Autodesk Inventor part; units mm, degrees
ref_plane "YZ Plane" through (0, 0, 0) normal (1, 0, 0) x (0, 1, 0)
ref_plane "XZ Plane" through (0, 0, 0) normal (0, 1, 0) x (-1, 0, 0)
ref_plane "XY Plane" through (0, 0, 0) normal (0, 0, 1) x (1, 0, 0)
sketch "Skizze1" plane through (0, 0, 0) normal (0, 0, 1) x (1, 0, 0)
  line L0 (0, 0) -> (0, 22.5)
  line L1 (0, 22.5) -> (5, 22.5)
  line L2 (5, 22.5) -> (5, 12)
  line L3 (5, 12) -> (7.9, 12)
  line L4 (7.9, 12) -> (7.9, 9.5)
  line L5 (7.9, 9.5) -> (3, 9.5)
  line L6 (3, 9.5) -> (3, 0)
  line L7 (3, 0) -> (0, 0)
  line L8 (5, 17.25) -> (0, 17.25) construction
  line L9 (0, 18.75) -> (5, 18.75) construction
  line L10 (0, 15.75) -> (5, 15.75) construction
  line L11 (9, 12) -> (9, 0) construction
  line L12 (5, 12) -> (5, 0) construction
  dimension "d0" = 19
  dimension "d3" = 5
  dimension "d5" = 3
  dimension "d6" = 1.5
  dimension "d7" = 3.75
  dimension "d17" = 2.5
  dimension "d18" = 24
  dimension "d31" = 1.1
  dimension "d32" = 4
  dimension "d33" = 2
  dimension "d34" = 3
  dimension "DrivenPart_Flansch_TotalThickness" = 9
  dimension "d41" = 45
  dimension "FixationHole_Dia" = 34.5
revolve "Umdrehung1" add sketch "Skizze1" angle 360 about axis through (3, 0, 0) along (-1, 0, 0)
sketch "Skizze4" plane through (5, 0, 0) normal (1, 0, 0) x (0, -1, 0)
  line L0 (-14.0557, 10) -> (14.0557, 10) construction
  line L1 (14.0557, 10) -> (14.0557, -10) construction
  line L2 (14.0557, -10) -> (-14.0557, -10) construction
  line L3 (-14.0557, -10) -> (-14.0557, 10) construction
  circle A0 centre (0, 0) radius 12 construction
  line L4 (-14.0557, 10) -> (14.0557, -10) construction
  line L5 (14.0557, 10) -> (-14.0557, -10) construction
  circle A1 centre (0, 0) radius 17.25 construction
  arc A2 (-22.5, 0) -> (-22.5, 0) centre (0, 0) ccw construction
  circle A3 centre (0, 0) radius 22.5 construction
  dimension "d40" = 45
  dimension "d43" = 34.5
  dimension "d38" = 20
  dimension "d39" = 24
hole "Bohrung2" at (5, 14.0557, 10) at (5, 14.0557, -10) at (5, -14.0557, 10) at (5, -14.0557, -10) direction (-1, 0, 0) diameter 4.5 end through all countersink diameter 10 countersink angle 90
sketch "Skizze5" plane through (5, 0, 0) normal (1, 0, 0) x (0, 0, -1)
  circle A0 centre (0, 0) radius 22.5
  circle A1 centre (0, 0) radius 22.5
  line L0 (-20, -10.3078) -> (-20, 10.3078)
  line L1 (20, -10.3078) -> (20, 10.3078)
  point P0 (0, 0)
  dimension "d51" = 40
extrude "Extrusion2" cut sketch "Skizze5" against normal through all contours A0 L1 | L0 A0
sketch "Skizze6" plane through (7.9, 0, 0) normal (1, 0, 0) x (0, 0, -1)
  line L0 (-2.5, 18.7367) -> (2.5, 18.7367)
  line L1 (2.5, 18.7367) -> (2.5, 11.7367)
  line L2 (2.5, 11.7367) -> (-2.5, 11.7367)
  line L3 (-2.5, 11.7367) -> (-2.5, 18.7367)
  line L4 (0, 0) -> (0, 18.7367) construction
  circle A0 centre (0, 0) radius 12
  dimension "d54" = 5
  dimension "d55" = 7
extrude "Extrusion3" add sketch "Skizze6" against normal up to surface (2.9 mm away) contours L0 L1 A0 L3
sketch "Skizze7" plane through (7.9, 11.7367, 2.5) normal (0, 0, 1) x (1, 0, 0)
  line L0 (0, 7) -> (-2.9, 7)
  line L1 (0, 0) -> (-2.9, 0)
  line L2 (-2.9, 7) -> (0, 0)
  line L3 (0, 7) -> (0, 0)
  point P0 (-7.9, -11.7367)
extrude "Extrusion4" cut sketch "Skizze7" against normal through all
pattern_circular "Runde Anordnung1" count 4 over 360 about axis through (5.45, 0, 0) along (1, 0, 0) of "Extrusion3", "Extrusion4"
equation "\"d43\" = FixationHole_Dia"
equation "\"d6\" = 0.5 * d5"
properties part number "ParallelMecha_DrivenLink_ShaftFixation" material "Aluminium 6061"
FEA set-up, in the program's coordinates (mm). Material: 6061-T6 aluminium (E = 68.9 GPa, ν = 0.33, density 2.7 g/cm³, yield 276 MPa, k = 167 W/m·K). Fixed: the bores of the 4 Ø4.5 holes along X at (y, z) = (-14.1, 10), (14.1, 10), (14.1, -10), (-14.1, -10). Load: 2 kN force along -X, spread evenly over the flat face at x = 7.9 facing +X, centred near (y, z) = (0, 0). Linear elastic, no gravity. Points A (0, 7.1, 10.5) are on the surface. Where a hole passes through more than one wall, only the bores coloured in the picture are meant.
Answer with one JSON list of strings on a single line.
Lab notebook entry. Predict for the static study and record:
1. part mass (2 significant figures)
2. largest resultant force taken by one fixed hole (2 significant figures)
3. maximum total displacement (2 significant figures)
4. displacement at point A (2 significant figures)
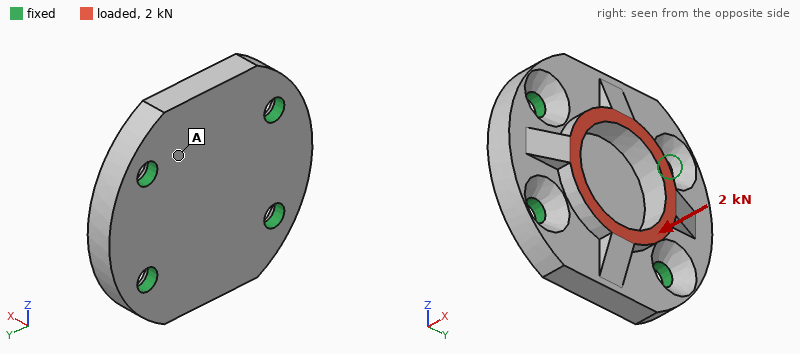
["19 g", "570 N", "9.0 µm", "5.6 µm"]
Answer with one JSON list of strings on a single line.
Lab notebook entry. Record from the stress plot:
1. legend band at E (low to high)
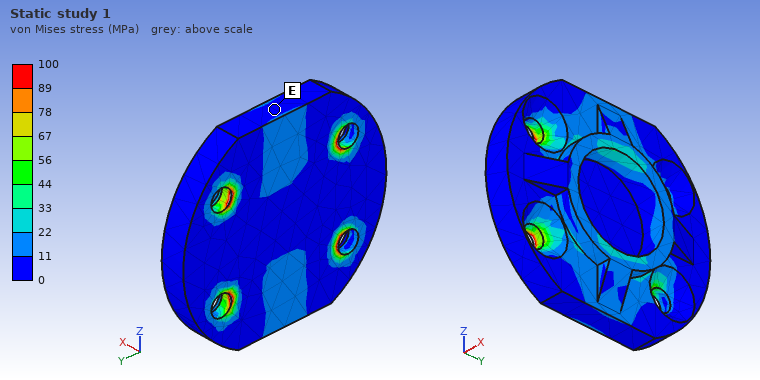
["0 to 11 MPa"]
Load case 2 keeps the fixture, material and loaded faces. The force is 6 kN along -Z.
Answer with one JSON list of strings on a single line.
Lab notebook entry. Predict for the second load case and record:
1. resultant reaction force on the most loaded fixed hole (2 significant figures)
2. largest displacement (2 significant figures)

["1.8 kN", "33 µm"]
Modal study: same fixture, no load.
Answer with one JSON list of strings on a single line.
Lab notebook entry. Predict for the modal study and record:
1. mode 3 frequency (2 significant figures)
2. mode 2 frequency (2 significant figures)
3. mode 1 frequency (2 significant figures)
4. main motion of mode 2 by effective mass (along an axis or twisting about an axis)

["29 kHz", "20 kHz", "19 kHz", "twisting about Y"]
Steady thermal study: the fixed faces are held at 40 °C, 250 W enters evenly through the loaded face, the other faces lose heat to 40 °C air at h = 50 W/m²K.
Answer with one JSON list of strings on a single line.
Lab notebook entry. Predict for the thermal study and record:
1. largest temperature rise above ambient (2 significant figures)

["73 K"]
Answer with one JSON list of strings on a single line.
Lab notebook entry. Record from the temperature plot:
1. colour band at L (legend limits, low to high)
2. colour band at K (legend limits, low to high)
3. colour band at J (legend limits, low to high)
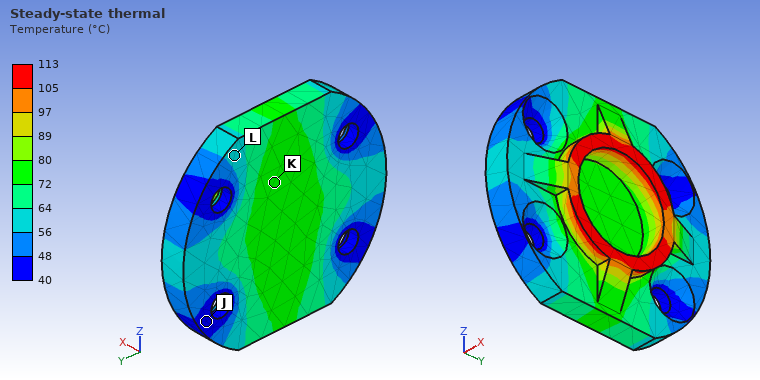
["56 to 64 °C", "72 to 80 °C", "40 to 48 °C"]
